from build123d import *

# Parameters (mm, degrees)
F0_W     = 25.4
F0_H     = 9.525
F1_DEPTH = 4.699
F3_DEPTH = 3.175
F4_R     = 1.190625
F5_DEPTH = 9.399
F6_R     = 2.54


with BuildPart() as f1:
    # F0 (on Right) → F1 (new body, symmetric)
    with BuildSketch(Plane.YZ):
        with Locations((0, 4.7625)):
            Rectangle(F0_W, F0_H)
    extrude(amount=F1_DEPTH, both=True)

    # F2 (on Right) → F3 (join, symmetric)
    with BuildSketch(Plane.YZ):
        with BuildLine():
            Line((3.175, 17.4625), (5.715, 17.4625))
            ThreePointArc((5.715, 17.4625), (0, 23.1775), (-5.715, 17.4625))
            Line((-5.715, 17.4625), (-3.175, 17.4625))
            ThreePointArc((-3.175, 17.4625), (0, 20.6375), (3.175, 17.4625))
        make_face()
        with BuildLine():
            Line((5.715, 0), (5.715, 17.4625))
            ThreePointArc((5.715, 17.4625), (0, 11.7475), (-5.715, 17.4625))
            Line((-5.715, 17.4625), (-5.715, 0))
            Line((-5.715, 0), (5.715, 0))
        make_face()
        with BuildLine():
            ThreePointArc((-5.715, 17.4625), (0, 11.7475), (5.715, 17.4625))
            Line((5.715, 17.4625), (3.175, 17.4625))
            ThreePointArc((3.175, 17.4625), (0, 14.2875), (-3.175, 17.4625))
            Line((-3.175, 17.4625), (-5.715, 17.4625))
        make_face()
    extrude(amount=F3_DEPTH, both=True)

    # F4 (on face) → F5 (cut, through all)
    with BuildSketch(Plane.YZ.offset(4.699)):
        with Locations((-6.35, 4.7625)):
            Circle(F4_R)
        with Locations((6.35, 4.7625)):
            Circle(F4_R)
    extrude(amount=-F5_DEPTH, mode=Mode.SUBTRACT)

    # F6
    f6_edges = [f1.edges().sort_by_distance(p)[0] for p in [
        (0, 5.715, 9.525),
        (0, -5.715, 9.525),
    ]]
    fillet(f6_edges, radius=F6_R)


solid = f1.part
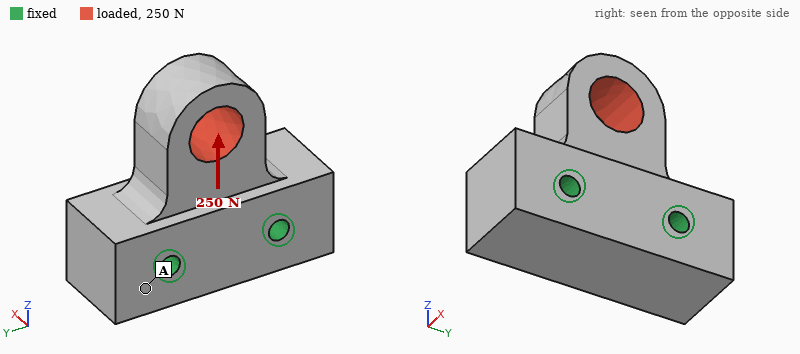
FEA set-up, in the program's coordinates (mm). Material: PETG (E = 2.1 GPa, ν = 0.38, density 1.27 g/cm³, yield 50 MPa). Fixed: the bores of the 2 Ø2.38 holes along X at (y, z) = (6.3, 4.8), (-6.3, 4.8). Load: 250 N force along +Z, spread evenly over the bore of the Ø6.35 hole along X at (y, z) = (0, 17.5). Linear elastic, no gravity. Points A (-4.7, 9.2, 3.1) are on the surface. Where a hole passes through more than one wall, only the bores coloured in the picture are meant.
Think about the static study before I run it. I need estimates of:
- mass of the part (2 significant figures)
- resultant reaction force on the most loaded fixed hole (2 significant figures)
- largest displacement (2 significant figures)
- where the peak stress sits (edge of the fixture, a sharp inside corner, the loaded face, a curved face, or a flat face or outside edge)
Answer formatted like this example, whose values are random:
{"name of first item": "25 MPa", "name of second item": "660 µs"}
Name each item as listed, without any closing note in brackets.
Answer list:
{"mass of the part": "3.7 g", "resultant reaction force on the most loaded fixed hole": "130 N", "largest displacement": "46 µm", "where the peak stress sits": "the loaded face"}
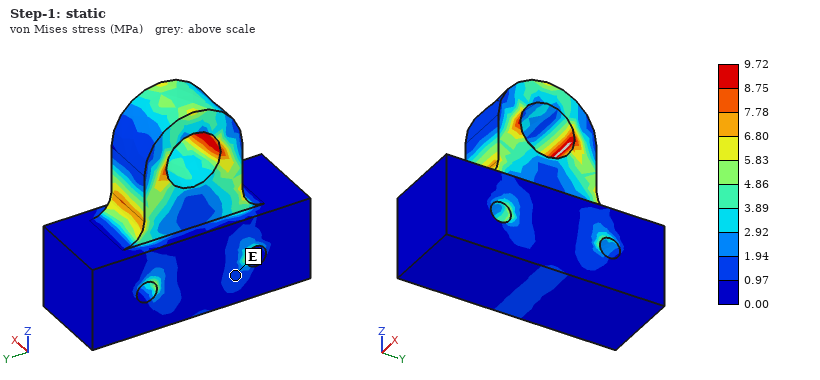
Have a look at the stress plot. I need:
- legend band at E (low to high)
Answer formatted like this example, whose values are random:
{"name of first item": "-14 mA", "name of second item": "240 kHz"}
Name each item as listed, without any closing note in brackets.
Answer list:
{"legend band at E": "0.97 to 1.94 MPa"}
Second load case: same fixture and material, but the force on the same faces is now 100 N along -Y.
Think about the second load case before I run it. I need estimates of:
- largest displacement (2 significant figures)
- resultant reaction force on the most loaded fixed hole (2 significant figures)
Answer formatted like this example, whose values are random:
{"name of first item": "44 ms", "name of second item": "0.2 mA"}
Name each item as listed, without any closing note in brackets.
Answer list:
{"largest displacement": "85 µm", "resultant reaction force on the most loaded fixed hole": "100 N"}
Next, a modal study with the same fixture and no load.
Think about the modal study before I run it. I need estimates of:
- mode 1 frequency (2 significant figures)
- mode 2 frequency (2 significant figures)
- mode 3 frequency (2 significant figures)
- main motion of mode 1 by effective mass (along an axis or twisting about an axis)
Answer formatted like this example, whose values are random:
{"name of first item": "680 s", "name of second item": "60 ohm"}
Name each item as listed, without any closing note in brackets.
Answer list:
{"mode 1 frequency": "5700 Hz", "mode 2 frequency": "8000 Hz", "mode 3 frequency": "11 kHz", "main motion of mode 1 by effective mass": "along X"}
